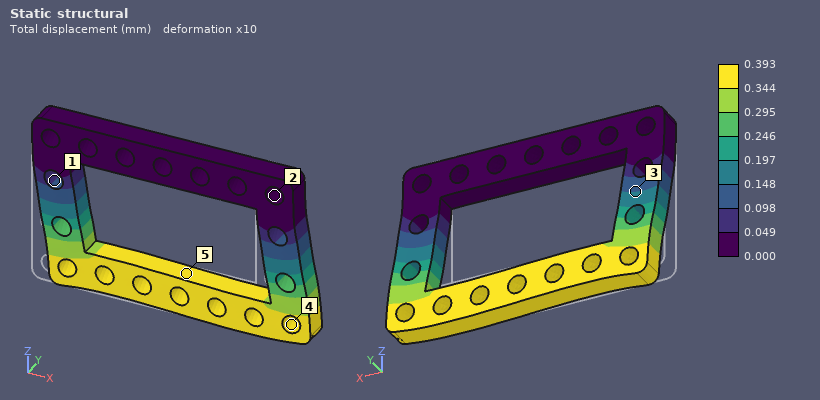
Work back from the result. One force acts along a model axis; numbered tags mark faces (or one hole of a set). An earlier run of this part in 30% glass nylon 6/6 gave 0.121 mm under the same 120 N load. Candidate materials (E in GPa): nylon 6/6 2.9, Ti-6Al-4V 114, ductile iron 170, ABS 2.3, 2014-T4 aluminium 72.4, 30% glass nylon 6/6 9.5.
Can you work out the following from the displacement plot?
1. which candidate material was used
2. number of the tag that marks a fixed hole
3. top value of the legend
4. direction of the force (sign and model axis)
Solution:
nylon 6/6
2
0.393 mm
+X
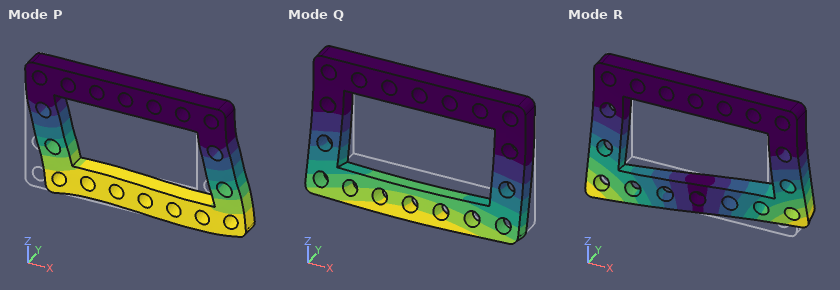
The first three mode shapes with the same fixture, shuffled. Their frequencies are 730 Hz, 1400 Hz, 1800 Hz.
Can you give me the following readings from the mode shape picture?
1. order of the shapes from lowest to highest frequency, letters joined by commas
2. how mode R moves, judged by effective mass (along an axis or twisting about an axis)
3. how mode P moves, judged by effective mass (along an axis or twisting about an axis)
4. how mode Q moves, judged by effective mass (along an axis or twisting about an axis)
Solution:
Q, R, P
twisting about Z
along X
along Y
